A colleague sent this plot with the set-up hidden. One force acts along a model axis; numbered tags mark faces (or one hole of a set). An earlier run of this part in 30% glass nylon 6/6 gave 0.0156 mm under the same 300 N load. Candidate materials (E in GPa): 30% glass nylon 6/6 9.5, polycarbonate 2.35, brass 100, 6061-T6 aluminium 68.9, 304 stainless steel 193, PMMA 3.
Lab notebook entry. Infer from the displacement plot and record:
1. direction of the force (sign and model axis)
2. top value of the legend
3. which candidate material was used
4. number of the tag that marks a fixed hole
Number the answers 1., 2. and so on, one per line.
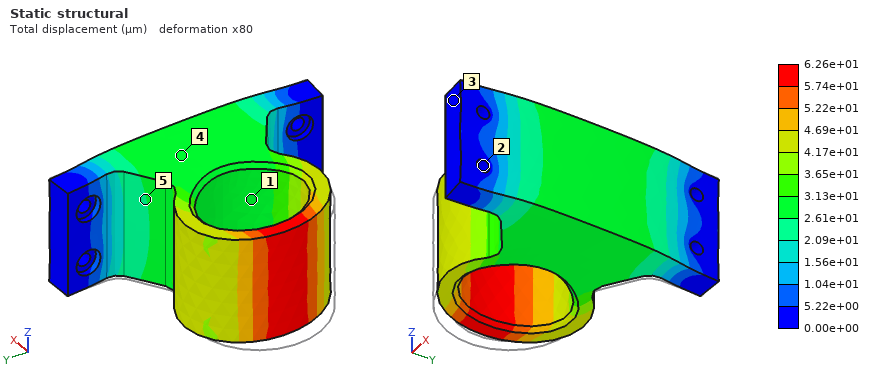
1. +X
2. 6.26e+01 µm
3. polycarbonate
4. 2
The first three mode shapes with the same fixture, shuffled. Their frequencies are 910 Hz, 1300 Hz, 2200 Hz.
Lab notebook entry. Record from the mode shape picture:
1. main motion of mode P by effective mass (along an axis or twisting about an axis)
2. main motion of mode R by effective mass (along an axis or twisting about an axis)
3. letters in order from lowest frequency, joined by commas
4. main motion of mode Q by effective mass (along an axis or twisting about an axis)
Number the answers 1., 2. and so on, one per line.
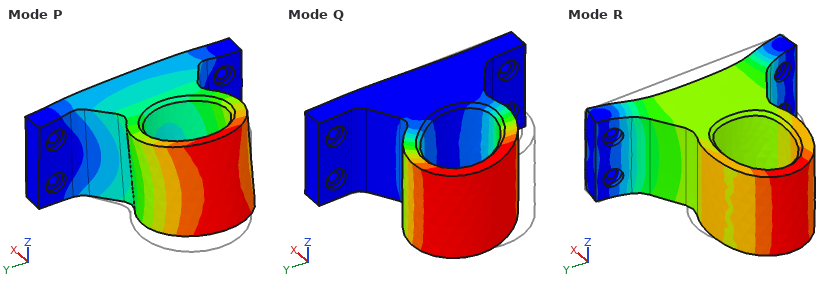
1. along Z
2. along X
3. P, Q, R
4. along Y
